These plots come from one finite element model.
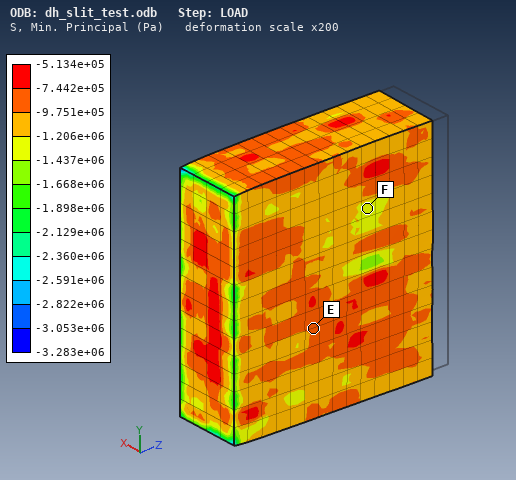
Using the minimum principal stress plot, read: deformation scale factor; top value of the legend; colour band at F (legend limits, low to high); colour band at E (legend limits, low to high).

200
-5.134e+05 Pa
-1.437e+06 to -1.206e+06 Pa
-9.751e+05 to -7.442e+05 Pa
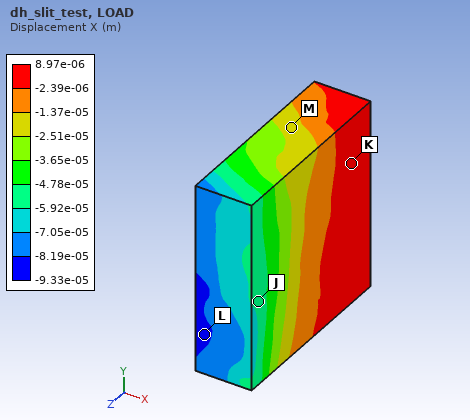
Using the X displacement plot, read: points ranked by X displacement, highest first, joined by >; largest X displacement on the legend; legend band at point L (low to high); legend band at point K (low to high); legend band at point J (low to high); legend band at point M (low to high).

K > M > J > L
8.97e-06 m
-9.33e-05 to -8.19e-05 m
-2.39e-06 to 8.97e-06 m
-5.92e-05 to -4.78e-05 m
-2.51e-05 to -1.37e-05 m
